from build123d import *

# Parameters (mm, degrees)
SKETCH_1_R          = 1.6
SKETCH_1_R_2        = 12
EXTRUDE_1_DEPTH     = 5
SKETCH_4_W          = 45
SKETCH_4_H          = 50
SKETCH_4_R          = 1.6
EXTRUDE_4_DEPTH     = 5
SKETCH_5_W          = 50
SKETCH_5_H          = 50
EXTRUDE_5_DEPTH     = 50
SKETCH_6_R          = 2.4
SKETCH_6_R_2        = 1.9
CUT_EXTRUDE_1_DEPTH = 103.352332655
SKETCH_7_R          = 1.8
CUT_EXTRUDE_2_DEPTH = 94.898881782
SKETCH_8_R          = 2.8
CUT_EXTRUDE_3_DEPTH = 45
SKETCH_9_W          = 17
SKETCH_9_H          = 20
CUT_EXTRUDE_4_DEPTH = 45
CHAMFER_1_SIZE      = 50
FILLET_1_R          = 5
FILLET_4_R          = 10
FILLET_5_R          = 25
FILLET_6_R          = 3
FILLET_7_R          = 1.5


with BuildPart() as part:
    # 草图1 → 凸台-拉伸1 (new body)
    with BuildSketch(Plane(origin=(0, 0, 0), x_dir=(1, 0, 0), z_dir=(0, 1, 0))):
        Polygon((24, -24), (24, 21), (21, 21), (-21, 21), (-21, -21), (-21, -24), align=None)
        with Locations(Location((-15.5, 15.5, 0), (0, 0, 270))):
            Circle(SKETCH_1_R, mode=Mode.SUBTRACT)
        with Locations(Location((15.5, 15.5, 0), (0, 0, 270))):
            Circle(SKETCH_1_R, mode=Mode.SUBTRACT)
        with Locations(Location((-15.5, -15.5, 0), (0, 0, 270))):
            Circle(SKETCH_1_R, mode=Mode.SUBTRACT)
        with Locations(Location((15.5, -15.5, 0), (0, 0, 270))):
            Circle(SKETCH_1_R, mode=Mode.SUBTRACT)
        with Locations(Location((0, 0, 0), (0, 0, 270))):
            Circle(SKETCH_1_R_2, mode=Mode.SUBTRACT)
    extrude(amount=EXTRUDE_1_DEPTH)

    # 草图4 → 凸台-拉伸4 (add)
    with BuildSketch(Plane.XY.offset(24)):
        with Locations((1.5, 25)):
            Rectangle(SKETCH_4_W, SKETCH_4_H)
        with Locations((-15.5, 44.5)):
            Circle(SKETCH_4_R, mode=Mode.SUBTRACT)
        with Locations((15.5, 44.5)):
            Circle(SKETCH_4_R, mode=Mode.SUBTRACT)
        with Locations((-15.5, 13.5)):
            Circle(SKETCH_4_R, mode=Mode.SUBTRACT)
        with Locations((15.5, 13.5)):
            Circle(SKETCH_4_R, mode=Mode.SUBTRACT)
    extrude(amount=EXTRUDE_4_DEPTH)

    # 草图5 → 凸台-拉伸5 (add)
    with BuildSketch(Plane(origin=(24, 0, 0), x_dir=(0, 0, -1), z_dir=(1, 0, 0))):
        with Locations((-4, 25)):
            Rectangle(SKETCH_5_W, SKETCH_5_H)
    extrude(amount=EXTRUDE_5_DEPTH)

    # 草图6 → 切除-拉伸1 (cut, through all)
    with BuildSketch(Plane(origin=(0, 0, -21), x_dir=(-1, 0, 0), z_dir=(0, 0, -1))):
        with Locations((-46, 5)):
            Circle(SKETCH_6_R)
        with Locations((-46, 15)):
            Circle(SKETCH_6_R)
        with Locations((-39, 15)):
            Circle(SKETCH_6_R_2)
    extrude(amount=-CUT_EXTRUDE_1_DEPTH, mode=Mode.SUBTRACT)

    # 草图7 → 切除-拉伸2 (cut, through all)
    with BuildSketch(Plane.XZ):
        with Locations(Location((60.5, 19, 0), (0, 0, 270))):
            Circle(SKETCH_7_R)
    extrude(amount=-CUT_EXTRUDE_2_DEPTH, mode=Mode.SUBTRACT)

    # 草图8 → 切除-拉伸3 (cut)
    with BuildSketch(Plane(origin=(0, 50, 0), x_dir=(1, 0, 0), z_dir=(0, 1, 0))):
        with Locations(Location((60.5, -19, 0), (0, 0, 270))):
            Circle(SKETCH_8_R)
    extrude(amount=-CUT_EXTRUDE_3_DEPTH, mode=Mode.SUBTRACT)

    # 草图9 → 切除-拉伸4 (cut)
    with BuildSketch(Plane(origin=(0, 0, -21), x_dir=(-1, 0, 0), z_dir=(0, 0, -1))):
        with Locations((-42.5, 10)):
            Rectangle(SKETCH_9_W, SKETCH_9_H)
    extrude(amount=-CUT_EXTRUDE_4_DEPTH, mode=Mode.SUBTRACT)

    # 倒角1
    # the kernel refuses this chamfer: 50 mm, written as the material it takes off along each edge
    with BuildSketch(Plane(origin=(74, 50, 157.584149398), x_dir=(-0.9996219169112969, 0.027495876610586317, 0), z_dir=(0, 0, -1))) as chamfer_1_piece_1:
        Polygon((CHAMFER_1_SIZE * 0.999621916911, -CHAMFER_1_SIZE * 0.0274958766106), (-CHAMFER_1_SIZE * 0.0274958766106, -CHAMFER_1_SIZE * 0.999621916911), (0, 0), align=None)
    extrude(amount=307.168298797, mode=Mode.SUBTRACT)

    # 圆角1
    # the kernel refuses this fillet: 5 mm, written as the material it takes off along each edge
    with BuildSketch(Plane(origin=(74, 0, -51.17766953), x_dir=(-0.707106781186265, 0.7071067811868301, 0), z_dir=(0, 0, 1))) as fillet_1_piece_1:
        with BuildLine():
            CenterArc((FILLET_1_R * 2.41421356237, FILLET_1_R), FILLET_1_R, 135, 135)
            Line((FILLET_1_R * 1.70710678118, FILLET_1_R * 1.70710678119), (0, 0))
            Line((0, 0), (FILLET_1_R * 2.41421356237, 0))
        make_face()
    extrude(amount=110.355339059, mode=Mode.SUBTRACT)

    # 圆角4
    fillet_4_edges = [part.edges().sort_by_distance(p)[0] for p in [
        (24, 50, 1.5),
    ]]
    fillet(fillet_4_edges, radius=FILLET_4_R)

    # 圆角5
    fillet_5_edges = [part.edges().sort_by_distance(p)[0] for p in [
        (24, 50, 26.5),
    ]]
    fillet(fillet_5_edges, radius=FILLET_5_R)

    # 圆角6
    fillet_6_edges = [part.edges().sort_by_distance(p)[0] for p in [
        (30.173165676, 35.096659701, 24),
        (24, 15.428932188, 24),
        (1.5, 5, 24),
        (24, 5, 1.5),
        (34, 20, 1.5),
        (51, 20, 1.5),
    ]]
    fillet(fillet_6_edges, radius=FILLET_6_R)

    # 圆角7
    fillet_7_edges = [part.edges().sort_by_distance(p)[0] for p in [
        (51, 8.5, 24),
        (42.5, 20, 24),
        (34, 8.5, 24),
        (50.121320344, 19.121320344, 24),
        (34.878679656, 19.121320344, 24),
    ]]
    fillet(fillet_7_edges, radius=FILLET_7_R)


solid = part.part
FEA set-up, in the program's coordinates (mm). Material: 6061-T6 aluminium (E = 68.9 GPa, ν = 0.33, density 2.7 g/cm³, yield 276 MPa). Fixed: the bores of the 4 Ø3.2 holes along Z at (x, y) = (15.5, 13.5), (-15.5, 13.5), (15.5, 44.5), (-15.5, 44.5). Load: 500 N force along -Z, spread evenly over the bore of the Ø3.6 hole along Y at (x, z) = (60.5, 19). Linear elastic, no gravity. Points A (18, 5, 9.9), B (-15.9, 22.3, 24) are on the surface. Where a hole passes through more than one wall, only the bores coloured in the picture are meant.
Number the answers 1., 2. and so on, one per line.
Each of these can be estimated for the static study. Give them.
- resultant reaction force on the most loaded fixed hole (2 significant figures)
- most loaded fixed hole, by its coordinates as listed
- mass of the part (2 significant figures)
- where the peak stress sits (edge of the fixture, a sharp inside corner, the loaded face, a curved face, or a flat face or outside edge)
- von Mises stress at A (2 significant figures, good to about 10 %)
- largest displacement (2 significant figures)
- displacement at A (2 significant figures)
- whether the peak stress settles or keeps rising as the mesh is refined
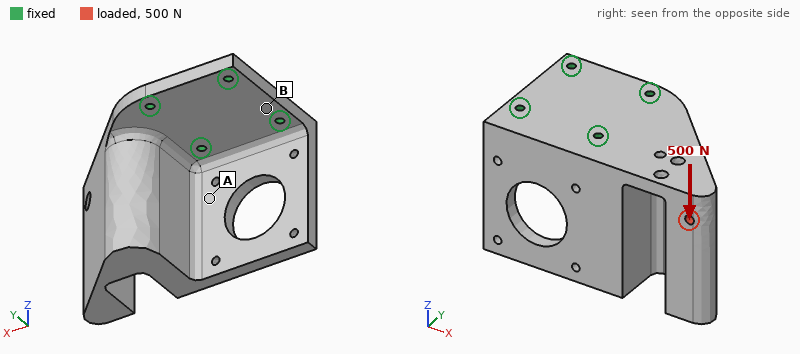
1. 1.3 kN
2. (15.5, 13.5)
3. 160 g
4. edge of the fixture
5. 11 MPa
6. 0.14 mm
7. 0.028 mm
8. keeps rising
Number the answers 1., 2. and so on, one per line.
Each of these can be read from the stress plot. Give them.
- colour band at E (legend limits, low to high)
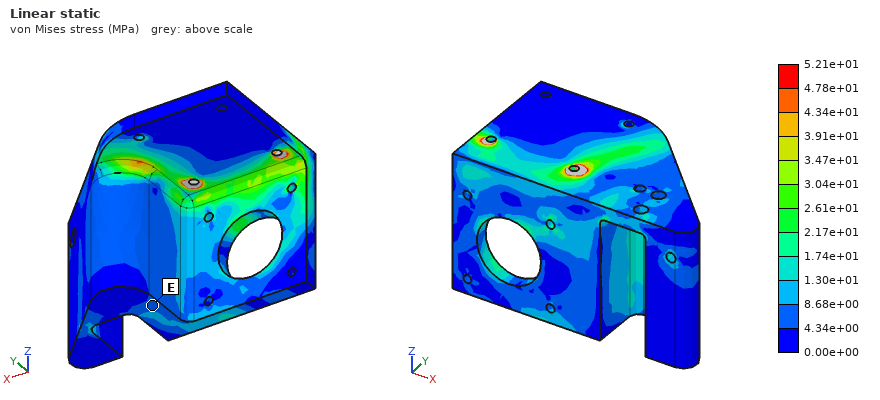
1. 4.34e+00 to 8.68e+00 MPa
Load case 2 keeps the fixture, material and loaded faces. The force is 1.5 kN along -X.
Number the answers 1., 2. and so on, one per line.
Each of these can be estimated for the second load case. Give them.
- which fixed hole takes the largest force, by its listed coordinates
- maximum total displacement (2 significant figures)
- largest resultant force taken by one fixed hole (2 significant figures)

1. (15.5, 13.5)
2. 82 µm
3. 1.3 kN
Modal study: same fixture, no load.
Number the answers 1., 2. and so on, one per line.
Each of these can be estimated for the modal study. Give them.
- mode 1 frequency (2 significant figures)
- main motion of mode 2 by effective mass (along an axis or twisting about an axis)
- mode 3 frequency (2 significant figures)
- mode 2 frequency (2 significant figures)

1. 1400 Hz
2. along Y
3. 3400 Hz
4. 2000 Hz
